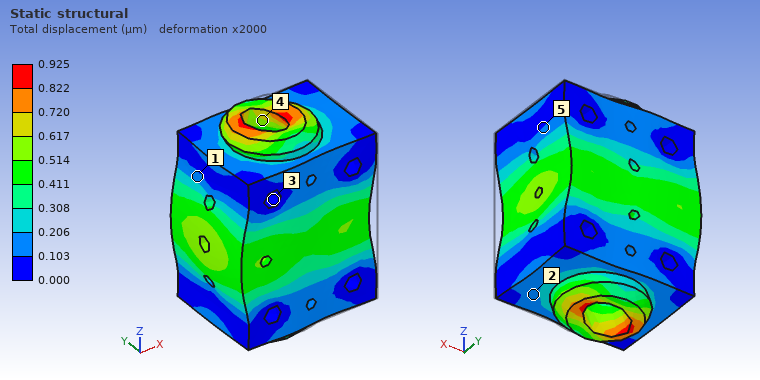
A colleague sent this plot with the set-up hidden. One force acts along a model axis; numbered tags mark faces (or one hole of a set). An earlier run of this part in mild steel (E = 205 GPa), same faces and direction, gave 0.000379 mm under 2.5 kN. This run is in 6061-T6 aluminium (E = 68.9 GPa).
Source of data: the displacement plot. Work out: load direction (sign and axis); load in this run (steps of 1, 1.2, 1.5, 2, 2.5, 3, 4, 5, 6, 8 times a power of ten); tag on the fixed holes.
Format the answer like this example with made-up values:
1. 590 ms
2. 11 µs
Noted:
1. -X
2. 2 kN
3. 3
